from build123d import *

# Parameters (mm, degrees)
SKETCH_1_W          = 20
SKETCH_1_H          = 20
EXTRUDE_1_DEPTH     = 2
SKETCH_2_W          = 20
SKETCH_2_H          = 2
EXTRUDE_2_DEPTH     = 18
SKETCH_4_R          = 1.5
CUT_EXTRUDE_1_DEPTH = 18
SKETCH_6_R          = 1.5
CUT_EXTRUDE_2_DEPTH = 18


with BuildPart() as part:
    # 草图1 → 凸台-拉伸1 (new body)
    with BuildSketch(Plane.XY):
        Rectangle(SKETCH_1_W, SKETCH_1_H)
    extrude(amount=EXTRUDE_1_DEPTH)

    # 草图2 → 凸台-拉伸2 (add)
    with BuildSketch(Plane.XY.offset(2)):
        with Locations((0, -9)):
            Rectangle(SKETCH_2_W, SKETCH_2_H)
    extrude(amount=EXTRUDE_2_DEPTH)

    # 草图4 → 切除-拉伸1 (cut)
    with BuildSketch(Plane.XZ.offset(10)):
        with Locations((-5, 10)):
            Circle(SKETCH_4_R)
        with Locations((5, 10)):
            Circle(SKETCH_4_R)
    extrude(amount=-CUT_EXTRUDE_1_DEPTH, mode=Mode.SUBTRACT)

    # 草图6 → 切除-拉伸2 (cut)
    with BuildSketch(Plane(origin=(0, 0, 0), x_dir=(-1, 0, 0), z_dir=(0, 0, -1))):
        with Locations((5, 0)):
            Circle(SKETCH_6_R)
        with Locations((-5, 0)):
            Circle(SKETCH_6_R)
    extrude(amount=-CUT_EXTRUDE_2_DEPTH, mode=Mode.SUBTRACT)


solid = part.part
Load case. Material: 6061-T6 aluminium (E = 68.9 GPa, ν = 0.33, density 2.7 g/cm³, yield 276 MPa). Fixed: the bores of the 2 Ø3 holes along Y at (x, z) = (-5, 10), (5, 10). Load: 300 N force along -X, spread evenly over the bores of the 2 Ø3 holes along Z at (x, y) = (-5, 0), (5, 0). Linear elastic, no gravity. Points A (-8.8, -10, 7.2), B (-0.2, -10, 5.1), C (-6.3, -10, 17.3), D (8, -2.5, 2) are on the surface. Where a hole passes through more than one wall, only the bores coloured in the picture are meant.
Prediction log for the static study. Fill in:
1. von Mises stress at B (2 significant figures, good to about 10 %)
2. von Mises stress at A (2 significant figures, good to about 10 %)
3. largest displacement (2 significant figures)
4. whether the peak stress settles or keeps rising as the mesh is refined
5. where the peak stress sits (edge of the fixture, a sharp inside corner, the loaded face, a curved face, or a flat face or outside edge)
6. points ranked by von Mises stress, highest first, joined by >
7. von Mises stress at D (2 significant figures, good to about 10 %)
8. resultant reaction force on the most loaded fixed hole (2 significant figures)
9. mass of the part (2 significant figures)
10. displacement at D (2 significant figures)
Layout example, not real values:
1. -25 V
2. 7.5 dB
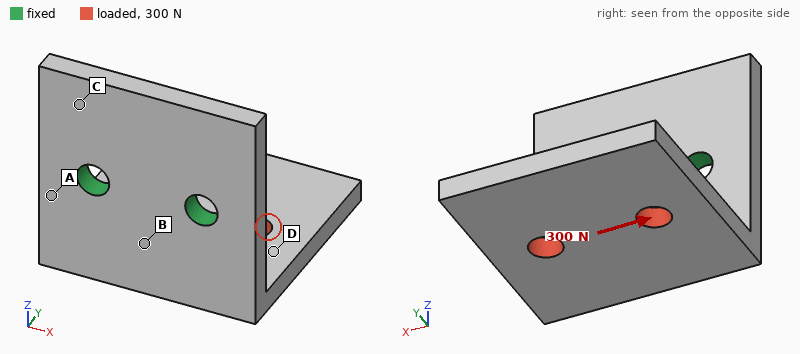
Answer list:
1. 58 MPa
2. 92 MPa
3. 0.15 mm
4. keeps rising
5. edge of the fixture
6. A > B > D > C
7. 35 MPa
8. 330 N
9. 4.0 g
10. 0.071 mm
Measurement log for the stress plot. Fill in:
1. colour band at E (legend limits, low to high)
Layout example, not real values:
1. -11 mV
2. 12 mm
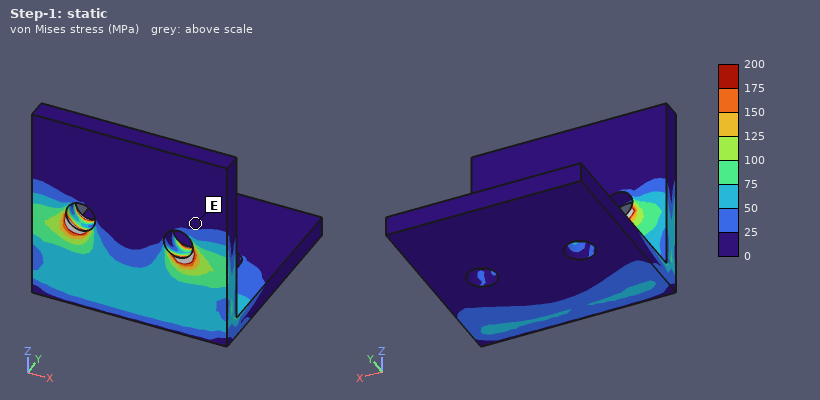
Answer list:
1. 0 to 25 MPa
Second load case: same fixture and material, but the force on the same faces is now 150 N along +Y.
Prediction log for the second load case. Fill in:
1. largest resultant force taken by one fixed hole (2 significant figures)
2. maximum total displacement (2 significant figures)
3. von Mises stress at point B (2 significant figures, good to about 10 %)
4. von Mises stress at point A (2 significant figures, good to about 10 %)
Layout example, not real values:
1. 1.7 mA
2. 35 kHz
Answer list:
1. 75 N
2. 0.11 mm
3. 40 MPa
4. 53 MPa
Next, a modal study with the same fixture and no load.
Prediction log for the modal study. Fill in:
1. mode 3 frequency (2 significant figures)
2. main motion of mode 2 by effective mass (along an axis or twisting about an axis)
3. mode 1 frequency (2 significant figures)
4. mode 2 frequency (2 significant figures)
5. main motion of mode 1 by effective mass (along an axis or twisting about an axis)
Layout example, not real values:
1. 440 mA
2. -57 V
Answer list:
1. 9700 Hz
2. along X
3. 2800 Hz
4. 5600 Hz
5. along Z
